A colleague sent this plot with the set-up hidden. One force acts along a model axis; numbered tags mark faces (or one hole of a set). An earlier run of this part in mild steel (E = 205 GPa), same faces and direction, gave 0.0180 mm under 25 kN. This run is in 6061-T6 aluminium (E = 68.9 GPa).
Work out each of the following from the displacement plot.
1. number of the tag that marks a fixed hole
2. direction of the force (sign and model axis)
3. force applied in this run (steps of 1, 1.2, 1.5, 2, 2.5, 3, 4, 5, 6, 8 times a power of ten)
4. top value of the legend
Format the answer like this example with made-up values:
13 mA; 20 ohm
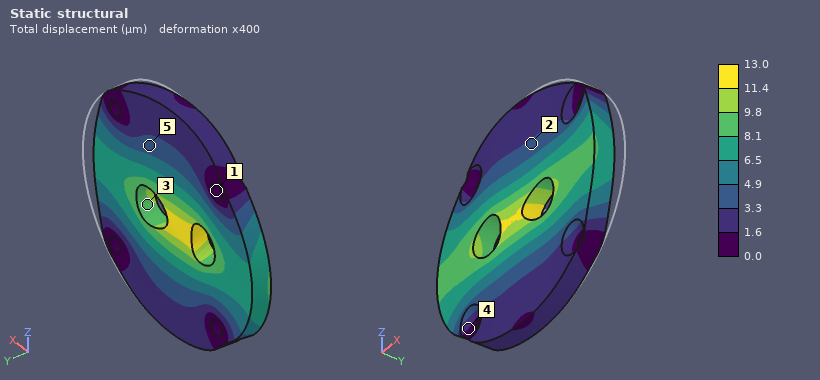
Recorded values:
1; -X; 6 kN; 13.0 µm
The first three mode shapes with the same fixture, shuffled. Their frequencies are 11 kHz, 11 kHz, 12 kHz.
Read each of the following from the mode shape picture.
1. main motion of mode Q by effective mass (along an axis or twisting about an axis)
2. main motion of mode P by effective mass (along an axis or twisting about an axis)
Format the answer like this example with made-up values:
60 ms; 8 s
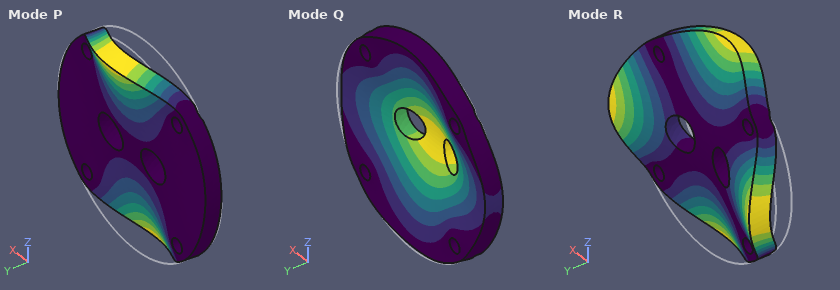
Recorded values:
along Y; twisting about X
